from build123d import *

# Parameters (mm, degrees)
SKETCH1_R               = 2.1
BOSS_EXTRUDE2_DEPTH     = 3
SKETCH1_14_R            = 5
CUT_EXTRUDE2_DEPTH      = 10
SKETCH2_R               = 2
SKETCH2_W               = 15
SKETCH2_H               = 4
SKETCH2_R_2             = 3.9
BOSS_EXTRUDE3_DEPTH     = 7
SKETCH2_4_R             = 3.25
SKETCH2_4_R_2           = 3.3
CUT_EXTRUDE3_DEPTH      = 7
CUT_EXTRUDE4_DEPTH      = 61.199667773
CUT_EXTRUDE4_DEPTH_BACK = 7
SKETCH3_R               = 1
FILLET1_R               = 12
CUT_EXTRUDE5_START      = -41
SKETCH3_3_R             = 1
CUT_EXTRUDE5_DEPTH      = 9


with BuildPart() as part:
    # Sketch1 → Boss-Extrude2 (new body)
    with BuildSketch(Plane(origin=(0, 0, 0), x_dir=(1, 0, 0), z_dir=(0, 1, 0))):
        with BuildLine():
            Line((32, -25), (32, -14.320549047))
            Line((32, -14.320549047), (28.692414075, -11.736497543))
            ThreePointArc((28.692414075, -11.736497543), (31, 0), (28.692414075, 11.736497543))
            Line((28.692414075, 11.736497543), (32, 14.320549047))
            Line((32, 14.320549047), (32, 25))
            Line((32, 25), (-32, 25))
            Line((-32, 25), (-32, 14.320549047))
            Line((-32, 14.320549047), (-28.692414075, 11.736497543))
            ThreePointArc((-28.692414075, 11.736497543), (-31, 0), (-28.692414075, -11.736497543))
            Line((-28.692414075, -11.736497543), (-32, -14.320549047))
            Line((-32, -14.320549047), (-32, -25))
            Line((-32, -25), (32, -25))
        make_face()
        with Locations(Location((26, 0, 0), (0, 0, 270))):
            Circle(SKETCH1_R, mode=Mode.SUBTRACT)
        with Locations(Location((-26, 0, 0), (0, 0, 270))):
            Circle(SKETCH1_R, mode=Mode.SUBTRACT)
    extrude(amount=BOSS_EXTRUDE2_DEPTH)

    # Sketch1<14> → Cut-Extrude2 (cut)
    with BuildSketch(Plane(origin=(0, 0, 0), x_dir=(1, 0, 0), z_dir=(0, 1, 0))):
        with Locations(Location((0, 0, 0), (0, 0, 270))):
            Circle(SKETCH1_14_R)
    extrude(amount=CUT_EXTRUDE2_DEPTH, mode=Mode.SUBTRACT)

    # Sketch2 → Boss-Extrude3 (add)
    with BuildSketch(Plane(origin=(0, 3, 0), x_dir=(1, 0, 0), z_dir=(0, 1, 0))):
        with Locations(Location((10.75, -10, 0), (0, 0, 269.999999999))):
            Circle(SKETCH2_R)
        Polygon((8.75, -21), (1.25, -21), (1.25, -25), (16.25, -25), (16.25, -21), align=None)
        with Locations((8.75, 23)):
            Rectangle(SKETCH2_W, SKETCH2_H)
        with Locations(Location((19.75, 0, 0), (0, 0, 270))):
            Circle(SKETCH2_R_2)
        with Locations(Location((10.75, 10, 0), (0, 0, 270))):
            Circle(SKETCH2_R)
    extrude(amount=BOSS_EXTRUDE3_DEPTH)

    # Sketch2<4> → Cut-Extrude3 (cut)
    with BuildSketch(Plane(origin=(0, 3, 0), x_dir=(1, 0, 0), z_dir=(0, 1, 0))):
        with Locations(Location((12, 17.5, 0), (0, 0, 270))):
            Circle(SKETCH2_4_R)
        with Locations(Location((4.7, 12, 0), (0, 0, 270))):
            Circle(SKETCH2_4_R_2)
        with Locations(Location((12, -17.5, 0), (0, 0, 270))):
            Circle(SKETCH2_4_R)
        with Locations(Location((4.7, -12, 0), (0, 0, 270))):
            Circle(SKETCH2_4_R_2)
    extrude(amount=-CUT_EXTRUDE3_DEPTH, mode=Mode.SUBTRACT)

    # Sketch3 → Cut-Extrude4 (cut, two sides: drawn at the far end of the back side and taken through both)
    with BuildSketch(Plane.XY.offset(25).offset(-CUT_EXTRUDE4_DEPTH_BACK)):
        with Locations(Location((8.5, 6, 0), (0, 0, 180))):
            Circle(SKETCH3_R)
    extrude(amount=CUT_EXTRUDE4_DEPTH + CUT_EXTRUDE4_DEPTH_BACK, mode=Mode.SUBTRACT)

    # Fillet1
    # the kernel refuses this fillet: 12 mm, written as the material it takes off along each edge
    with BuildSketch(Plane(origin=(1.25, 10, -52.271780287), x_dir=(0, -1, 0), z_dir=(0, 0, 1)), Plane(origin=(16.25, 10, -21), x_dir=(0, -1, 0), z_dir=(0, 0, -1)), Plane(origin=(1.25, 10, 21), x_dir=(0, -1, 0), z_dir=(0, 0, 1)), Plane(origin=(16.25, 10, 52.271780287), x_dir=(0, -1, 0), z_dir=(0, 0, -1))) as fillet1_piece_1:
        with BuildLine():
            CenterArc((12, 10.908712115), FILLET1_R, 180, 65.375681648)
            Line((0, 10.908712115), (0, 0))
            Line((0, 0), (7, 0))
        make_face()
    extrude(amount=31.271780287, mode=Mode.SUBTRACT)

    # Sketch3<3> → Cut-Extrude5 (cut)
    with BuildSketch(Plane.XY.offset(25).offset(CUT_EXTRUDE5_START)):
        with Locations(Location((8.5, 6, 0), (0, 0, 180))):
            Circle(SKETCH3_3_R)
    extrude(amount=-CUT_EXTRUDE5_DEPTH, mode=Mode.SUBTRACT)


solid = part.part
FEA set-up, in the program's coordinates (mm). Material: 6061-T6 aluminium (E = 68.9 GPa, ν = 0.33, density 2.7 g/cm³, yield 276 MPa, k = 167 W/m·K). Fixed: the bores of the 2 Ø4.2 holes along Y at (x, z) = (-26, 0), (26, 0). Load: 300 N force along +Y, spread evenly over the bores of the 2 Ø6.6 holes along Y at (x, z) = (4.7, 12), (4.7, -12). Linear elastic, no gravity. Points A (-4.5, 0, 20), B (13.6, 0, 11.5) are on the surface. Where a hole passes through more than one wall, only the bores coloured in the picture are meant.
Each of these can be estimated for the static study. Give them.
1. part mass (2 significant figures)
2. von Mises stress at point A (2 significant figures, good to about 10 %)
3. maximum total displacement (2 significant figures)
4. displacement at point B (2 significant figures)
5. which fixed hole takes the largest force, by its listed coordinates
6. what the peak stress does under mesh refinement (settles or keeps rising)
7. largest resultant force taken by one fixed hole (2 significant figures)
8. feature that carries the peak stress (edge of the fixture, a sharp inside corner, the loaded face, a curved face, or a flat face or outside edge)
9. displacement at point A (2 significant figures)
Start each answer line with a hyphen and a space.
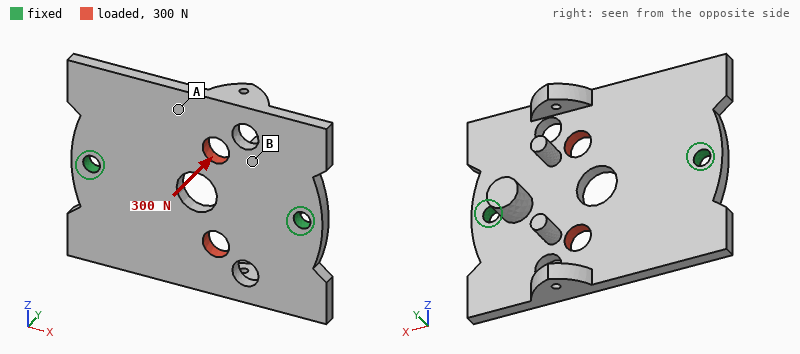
- 26 g
- 16 MPa
- 57 µm
- 31 µm
- (26, 0)
- keeps rising
- 190 N
- edge of the fixture
- 50 µm
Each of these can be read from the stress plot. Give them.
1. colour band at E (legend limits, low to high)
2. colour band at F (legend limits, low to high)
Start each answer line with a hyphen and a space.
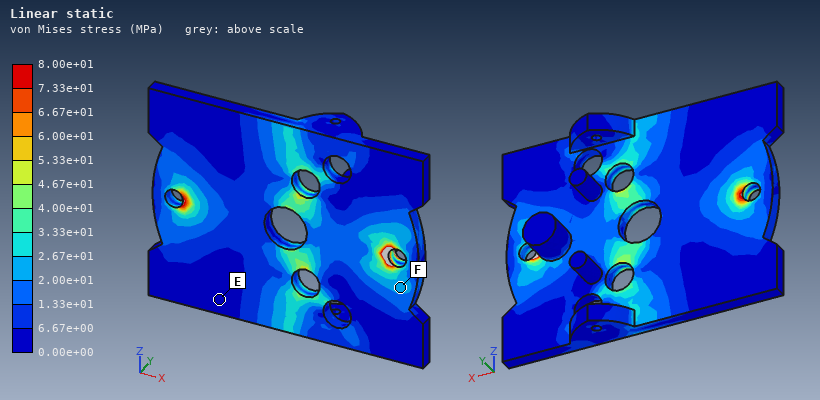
- 0.00e+00 to 6.67e+00 MPa
- 2.00e+01 to 2.67e+01 MPa
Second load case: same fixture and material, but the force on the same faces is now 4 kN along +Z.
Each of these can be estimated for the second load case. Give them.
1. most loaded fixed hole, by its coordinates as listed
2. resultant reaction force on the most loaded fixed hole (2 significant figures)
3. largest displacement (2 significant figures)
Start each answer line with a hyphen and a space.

- (26, 0)
- 2.4 kN
- 27 µm
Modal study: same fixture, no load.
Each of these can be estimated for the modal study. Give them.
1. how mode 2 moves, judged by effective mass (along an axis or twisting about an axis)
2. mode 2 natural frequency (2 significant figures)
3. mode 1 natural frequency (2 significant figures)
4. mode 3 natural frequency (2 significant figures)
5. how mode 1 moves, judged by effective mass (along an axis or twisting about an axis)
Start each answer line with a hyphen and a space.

- along Y
- 3200 Hz
- 2400 Hz
- 4900 Hz
- twisting about X
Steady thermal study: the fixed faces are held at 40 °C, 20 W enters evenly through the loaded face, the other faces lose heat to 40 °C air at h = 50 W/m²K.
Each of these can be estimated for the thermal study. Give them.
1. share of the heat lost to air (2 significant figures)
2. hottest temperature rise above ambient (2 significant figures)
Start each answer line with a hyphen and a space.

- 15 %
- 15 K
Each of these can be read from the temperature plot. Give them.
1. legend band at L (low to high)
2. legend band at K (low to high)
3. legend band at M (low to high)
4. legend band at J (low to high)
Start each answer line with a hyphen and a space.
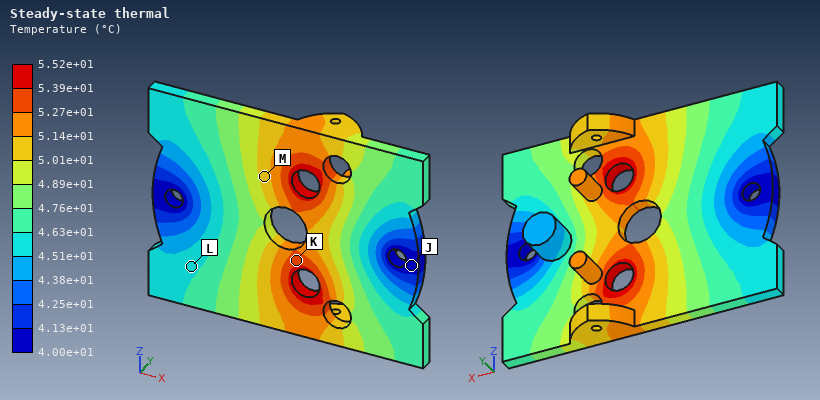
- 4.51e+01 to 4.63e+01 °C
- 5.27e+01 to 5.39e+01 °C
- 5.01e+01 to 5.14e+01 °C
- 4.00e+01 to 4.13e+01 °C
